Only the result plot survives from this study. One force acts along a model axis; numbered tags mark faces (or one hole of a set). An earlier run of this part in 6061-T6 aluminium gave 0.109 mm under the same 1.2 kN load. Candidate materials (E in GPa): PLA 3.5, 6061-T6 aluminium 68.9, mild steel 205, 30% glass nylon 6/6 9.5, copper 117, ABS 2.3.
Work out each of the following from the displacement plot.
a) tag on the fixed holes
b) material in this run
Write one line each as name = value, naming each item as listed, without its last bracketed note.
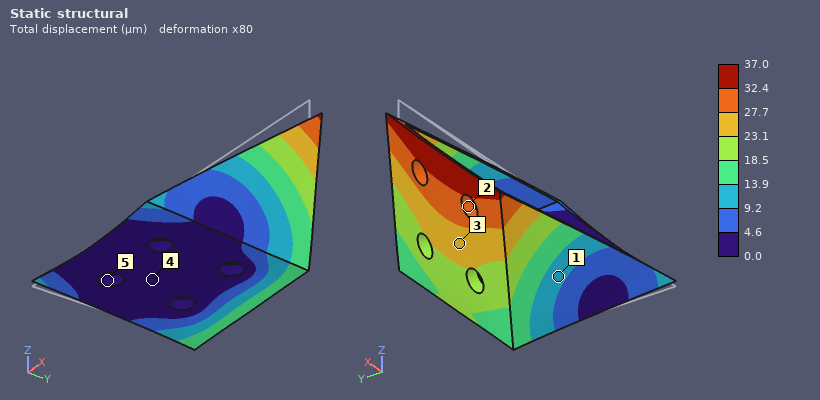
tag on the fixed holes = 5
material in this run = mild steel
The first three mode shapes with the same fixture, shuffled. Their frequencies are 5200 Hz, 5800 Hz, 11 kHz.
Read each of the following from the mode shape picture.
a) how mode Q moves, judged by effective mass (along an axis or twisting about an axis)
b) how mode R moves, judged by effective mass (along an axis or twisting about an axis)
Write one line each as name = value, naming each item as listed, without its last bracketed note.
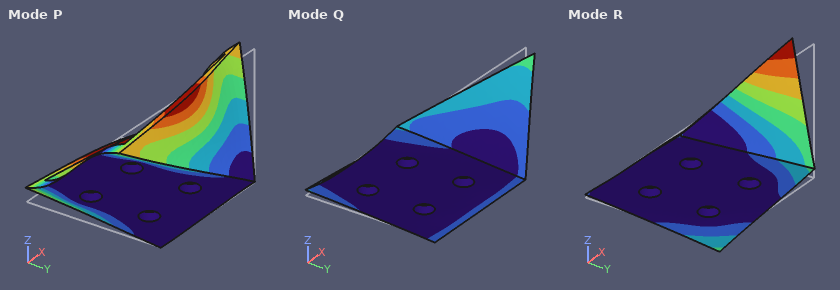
how mode Q moves, judged by effective mass = along Y
how mode R moves, judged by effective mass = along X
